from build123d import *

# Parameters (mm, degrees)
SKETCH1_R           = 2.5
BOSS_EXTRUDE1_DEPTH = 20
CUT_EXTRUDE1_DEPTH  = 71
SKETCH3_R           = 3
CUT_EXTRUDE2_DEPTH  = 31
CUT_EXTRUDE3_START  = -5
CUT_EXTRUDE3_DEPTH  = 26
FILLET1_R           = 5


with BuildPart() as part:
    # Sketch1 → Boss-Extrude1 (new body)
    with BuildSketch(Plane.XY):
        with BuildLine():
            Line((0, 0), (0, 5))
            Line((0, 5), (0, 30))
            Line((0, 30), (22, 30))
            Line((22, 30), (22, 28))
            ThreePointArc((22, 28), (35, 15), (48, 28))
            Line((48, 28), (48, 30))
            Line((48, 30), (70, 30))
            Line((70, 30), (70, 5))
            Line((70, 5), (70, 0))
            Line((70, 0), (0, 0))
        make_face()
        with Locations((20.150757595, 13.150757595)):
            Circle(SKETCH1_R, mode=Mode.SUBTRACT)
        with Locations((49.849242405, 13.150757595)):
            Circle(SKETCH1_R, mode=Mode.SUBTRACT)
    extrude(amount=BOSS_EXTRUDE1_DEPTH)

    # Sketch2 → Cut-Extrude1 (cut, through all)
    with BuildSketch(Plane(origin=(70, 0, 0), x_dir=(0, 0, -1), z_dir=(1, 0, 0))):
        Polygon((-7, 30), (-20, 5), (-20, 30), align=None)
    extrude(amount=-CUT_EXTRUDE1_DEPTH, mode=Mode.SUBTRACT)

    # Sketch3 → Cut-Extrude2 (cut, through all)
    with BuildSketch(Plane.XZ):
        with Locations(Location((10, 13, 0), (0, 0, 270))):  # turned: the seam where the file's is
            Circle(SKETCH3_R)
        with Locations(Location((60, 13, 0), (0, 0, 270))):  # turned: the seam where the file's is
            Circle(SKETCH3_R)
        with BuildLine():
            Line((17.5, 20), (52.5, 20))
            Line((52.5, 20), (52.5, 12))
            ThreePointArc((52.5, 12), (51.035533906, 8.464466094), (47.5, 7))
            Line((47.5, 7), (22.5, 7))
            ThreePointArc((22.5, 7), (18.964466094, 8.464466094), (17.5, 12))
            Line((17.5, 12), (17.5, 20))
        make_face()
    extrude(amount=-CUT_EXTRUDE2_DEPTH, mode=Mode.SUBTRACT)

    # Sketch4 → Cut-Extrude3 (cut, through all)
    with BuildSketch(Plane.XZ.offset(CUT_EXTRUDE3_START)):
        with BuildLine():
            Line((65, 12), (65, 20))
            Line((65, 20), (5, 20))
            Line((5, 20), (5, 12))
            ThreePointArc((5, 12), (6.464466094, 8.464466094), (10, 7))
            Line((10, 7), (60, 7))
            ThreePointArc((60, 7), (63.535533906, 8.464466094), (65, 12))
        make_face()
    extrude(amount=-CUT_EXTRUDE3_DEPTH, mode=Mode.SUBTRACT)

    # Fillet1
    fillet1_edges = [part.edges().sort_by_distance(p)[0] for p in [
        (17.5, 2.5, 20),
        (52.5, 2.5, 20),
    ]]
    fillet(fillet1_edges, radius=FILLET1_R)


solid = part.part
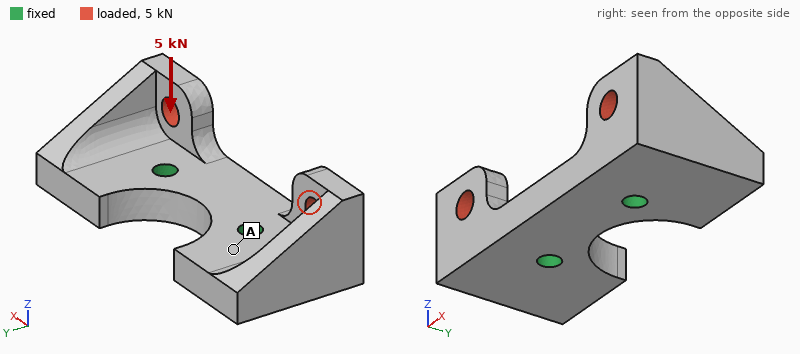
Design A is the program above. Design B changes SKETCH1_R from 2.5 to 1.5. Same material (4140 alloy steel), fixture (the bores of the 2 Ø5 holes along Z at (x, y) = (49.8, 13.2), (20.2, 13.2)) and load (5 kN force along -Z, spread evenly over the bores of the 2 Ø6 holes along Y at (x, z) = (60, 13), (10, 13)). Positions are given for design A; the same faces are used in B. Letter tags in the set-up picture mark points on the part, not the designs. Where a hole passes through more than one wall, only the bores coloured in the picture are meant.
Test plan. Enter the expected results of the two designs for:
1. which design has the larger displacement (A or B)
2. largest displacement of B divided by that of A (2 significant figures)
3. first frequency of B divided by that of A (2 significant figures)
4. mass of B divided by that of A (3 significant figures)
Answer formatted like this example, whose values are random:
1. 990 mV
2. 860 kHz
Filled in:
1. B
2. 1.3
3. 0.86
4. 1.01
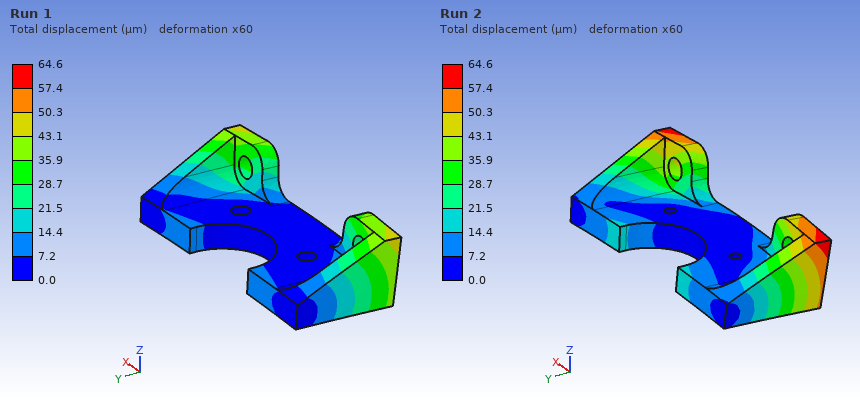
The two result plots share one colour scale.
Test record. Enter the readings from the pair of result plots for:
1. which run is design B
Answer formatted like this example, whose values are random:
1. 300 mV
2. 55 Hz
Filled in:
1. Run 2
